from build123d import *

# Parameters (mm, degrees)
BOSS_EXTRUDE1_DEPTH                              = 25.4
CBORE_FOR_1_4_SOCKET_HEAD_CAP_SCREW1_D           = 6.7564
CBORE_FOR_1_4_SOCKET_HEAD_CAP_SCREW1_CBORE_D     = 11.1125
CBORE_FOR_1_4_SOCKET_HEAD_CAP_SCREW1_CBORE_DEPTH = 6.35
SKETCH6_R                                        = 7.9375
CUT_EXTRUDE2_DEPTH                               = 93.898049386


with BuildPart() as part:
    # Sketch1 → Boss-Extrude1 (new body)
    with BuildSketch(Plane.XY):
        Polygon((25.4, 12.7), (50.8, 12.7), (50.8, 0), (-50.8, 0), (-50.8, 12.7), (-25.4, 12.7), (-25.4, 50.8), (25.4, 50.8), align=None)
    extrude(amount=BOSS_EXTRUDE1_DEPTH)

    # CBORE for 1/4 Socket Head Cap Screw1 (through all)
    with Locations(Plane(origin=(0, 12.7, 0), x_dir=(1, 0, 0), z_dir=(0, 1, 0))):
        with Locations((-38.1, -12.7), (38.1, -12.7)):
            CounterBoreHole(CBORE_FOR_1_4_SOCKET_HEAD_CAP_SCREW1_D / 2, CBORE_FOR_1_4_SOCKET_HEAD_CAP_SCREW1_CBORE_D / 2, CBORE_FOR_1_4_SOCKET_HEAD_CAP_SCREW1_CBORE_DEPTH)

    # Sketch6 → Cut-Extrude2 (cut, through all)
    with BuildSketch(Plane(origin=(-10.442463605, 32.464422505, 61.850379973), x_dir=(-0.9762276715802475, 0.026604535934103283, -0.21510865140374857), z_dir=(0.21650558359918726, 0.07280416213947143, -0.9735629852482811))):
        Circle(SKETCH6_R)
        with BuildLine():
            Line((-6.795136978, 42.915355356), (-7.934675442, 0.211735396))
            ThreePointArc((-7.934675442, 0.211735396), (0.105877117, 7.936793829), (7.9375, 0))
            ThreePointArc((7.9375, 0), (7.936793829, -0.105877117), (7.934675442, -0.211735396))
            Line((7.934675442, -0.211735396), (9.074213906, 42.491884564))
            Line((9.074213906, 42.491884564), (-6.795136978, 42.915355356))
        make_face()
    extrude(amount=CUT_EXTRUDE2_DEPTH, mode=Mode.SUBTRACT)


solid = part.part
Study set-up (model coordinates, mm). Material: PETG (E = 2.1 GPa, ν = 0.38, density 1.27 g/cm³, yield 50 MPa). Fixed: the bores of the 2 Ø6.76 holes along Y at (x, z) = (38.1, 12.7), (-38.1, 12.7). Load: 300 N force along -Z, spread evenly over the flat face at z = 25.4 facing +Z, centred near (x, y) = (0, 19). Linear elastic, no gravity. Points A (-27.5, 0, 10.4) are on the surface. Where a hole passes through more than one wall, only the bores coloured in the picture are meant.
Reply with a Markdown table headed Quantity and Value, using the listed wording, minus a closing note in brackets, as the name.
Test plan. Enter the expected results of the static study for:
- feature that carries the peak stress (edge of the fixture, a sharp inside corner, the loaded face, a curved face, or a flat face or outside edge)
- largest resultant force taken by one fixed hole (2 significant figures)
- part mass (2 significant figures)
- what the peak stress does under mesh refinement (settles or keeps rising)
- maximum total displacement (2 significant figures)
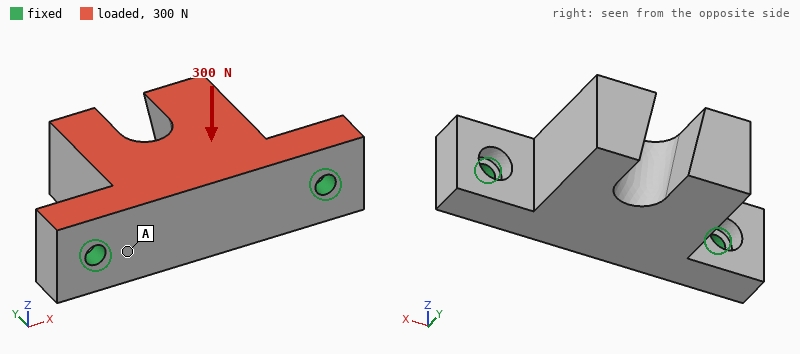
| Quantity | Value |
|---|---|
| feature that carries the peak stress | edge of the fixture |
| largest resultant force taken by one fixed hole | 150 N |
| part mass | 91 g |
| what the peak stress does under mesh refinement | keeps rising |
| maximum total displacement | 0.39 mm |
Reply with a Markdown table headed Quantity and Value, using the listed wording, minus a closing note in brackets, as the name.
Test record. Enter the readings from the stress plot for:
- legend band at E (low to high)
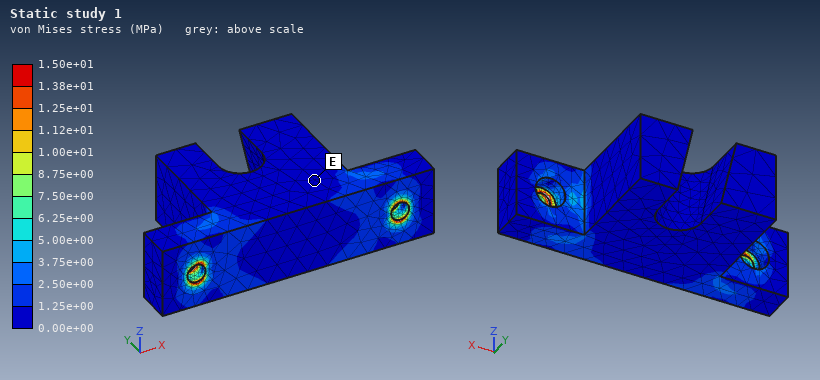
| Quantity | Value |
|---|---|
| legend band at E | 0.00e+00 to 1.25e+00 MPa |
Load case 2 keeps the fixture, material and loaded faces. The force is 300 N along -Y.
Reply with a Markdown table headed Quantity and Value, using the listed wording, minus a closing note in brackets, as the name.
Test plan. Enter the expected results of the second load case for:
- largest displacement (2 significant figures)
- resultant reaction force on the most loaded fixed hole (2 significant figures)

| Quantity | Value |
|---|---|
| largest displacement | 0.28 mm |
| resultant reaction force on the most loaded fixed hole | 180 N |
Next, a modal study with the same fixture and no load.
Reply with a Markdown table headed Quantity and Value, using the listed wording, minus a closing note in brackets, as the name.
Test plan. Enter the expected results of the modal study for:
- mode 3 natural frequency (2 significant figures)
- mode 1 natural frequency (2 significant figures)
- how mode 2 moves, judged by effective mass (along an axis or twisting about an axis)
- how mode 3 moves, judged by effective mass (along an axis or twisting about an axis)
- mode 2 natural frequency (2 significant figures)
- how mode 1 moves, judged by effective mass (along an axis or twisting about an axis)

| Quantity | Value |
|---|---|
| mode 3 natural frequency | 2000 Hz |
| mode 1 natural frequency | 570 Hz |
| how mode 2 moves, judged by effective mass | along Y |
| how mode 3 moves, judged by effective mass | along X |
| mode 2 natural frequency | 1800 Hz |
| how mode 1 moves, judged by effective mass | along Z |
